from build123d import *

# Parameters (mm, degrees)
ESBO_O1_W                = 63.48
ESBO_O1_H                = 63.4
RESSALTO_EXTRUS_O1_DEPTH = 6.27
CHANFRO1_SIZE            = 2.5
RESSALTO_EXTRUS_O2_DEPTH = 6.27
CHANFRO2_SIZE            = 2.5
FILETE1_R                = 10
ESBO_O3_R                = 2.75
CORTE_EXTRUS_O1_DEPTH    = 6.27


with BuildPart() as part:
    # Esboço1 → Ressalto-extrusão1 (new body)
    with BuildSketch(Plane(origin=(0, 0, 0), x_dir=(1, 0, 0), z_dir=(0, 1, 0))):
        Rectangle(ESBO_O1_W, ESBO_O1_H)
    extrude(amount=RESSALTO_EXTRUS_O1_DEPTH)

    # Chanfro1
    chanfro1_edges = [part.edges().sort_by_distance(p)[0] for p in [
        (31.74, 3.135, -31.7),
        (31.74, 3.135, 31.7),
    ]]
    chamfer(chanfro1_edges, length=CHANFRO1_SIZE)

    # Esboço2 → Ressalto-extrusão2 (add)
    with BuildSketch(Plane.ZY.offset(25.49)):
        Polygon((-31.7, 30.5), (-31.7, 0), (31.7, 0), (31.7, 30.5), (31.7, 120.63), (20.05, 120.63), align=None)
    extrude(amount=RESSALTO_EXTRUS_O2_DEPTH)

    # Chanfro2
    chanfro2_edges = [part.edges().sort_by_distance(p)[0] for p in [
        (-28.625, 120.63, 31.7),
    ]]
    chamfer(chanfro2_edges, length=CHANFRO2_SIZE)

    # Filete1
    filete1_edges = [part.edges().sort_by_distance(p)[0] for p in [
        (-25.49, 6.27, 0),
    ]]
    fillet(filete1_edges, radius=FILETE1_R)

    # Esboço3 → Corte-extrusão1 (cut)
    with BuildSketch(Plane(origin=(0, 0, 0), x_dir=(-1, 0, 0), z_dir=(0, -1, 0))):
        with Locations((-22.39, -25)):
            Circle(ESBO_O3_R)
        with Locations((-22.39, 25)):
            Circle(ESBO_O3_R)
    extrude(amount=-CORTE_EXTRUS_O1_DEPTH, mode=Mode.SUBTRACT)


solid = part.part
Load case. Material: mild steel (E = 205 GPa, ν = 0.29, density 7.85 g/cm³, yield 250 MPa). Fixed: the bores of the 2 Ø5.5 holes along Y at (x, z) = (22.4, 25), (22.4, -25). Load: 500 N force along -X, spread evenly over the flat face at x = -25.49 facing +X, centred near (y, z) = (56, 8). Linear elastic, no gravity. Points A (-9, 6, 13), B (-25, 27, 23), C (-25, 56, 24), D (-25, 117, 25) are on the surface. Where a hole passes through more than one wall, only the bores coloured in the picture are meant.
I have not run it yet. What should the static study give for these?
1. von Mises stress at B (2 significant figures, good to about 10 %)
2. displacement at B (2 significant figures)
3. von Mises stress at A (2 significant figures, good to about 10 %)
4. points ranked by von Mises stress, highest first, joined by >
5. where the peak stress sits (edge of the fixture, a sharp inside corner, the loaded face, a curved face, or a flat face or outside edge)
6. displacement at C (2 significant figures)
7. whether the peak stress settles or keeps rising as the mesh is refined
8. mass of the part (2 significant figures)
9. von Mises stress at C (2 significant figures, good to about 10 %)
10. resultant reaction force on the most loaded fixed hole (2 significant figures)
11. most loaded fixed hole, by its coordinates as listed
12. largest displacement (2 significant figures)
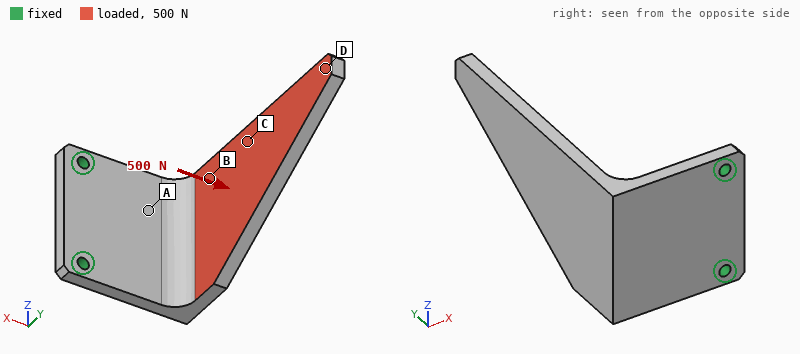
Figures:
38 MPa
0.18 mm
62 MPa
A > B > C > D
edge of the fixture
0.34 mm
keeps rising
450 g
20 MPa
340 N
(22.4, 25)
0.84 mm
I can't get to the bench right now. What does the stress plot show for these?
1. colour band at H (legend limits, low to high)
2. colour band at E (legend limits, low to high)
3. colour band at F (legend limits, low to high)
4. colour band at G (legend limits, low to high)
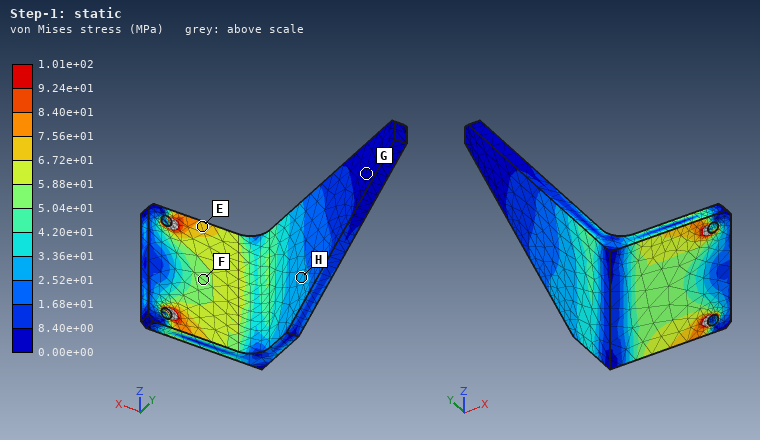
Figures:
2.52e+01 to 3.36e+01 MPa
6.72e+01 to 7.56e+01 MPa
5.04e+01 to 5.88e+01 MPa
0.00e+00 to 8.40e+00 MPa
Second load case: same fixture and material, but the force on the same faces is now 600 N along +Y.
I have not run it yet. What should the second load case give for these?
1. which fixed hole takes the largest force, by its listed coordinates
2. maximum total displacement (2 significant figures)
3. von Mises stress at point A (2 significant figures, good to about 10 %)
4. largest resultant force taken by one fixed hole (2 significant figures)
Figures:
(22.4, 25)
0.33 mm
24 MPa
390 N
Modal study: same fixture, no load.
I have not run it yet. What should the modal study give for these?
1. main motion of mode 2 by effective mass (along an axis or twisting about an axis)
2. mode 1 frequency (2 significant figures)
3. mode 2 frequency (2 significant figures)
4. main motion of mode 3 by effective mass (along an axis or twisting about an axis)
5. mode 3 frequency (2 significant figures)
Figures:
along Z
330 Hz
700 Hz
along Y
1000 Hz
